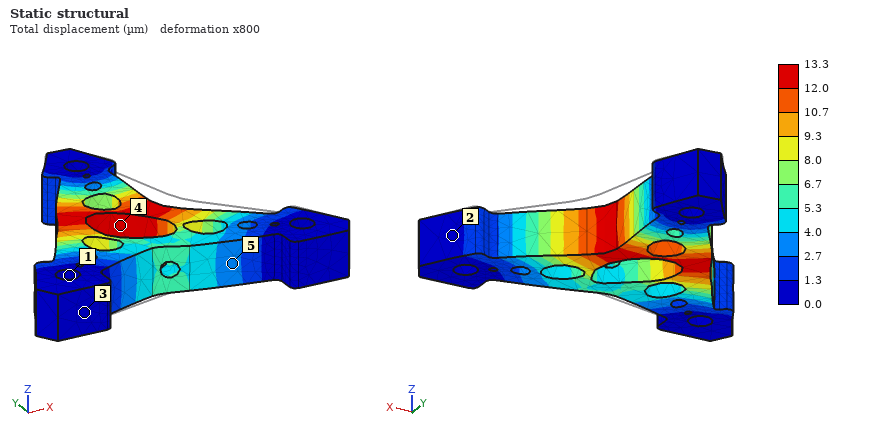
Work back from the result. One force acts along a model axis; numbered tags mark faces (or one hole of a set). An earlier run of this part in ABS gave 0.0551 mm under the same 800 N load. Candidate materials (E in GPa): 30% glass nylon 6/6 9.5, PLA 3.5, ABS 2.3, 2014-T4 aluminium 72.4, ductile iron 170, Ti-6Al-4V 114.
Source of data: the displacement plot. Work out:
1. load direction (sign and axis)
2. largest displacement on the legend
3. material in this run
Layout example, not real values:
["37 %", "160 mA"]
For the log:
["-X", "13.3 µm", "30% glass nylon 6/6"]
